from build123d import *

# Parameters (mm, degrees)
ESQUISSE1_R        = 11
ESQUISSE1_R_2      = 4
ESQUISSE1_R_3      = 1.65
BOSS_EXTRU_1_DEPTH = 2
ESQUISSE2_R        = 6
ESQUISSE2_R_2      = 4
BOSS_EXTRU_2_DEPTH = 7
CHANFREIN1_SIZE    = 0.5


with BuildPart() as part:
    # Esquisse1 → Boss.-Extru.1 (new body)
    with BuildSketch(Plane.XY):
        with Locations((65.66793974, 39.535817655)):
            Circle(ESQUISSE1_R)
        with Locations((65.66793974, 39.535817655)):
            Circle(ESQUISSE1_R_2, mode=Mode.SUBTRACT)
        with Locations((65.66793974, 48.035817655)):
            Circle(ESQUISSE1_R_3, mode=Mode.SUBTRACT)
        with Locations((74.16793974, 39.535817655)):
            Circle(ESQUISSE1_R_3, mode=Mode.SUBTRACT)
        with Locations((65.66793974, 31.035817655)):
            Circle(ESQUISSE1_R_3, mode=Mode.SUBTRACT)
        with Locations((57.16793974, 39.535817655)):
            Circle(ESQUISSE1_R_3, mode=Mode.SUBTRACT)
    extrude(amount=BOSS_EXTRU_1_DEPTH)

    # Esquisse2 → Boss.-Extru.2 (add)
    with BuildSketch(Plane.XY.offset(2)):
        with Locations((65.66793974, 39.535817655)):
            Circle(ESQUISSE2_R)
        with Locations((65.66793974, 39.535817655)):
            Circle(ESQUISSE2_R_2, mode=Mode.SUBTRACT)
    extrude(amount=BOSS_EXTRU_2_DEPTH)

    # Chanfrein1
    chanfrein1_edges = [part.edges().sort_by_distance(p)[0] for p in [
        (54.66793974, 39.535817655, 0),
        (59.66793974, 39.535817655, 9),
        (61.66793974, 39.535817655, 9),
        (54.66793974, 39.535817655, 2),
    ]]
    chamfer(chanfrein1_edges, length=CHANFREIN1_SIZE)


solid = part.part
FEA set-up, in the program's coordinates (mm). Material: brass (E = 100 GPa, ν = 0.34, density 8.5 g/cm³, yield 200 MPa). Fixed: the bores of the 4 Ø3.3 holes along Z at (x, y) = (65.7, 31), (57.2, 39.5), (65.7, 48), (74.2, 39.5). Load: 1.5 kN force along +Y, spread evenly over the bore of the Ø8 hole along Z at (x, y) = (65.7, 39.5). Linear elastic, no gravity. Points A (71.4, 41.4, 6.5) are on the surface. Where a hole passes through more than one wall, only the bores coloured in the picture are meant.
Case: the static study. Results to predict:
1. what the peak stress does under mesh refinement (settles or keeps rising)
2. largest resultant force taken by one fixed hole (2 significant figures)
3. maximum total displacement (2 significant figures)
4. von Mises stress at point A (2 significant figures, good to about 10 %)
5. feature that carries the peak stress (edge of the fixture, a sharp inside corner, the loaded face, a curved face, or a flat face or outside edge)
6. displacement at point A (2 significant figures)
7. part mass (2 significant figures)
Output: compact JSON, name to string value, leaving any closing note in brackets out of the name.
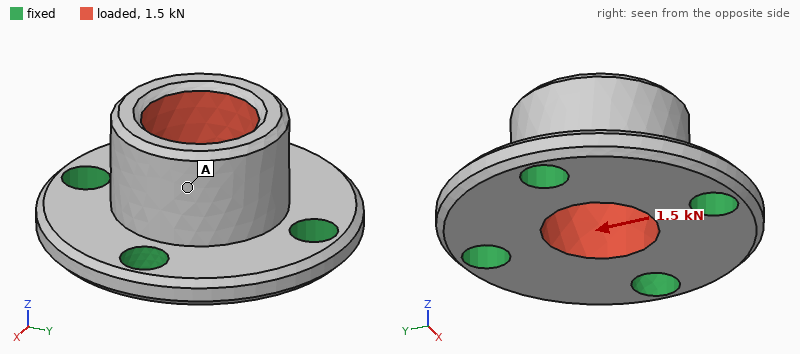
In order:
{"what the peak stress does under mesh refinement": "keeps rising", "largest resultant force taken by one fixed hole": "560 N", "maximum total displacement": "7.6 µm", "von Mises stress at point A": "15 MPa", "feature that carries the peak stress": "edge of the fixture", "displacement at point A": "5.1 µm", "part mass": "8.6 g"}
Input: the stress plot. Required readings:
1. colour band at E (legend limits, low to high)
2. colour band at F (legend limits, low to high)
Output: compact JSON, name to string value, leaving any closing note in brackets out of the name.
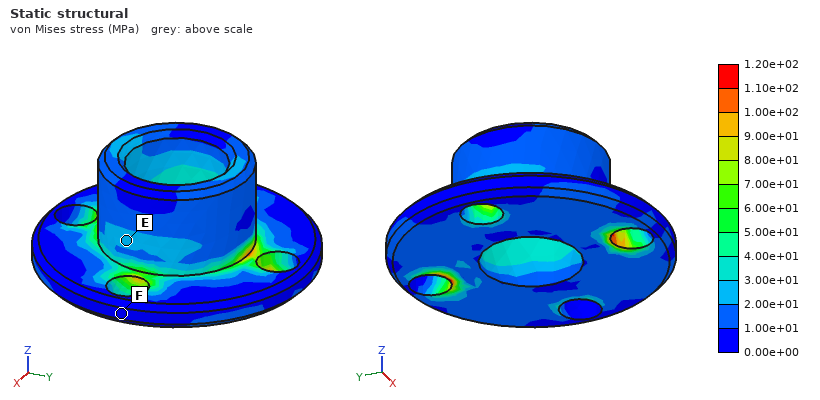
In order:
{"colour band at E": "2.00e+01 to 3.00e+01 MPa", "colour band at F": "0.00e+00 to 1.00e+01 MPa"}
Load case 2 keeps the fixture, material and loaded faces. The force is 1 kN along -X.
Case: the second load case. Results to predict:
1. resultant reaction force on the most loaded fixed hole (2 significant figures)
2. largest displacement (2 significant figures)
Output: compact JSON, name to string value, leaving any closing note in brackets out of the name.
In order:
{"resultant reaction force on the most loaded fixed hole": "370 N", "largest displacement": "5.1 µm"}
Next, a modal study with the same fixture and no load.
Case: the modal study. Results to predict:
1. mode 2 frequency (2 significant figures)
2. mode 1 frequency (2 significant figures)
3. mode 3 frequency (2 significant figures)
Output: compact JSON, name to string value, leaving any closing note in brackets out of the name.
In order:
{"mode 2 frequency": "35 kHz", "mode 1 frequency": "35 kHz", "mode 3 frequency": "40 kHz"}
